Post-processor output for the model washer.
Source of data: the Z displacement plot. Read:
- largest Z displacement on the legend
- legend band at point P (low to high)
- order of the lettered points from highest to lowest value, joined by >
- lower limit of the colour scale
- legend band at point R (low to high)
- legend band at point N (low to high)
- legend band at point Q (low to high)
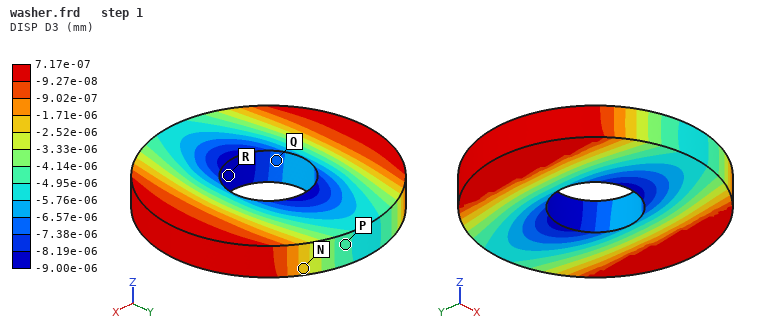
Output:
7.17e-07 mm
-4.95e-06 to -4.14e-06 mm
N > P > Q > R
-9.00e-06 mm
-9.00e-06 to -8.19e-06 mm
-2.52e-06 to -1.71e-06 mm
-7.38e-06 to -6.57e-06 mm
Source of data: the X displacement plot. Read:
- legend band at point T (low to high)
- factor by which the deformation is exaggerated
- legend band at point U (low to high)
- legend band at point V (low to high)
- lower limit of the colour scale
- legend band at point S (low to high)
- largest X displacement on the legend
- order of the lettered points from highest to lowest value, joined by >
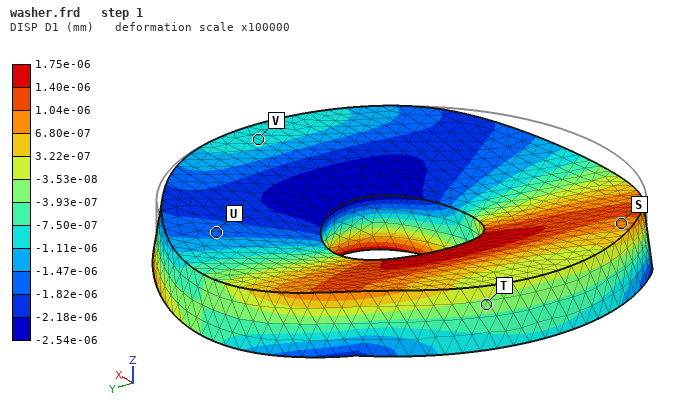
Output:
-3.93e-07 to -3.53e-08 mm
100000
-1.82e-06 to -1.47e-06 mm
-1.11e-06 to -7.50e-07 mm
-2.54e-06 mm
6.80e-07 to 1.04e-06 mm
1.75e-06 mm
S > T > V > U
